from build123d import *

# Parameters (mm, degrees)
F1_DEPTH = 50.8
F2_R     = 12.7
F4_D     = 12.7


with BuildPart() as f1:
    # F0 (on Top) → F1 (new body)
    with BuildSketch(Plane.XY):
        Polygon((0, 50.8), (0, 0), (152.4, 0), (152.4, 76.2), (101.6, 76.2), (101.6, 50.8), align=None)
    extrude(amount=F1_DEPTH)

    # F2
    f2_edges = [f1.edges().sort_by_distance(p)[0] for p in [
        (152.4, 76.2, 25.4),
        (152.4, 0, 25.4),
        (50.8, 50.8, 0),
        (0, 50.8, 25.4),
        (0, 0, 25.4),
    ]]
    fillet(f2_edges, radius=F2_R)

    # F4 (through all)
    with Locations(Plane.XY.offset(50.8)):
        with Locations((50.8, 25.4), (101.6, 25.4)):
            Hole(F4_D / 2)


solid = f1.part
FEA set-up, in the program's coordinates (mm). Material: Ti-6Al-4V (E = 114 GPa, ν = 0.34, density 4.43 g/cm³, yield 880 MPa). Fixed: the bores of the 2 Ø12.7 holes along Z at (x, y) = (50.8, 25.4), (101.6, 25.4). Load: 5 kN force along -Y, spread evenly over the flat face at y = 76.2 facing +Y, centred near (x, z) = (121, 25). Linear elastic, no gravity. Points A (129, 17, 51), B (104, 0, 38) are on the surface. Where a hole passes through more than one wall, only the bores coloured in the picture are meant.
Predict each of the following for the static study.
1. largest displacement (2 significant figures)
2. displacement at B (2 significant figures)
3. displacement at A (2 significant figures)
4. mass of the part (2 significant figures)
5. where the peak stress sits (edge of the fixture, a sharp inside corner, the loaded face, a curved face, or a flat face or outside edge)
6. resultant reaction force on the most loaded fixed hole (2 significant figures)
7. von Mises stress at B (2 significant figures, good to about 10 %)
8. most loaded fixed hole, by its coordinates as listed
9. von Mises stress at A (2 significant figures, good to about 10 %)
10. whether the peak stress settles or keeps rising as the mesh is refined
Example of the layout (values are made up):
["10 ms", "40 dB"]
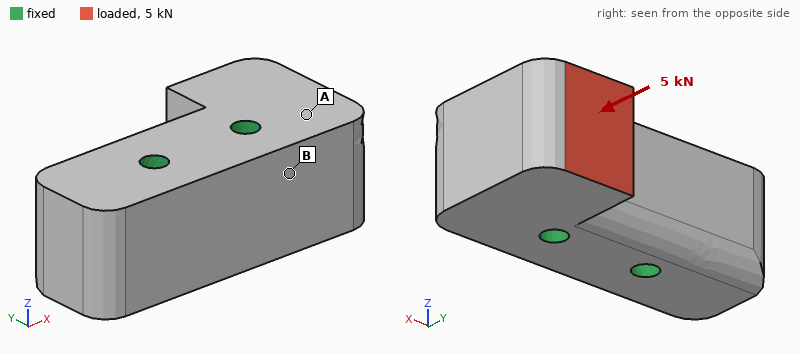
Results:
["4.2 µm", "0.85 µm", "1.8 µm", "1.9 kg", "edge of the fixture", "6.0 kN", "3.4 MPa", "(101.6, 25.4)", "1.5 MPa", "keeps rising"]
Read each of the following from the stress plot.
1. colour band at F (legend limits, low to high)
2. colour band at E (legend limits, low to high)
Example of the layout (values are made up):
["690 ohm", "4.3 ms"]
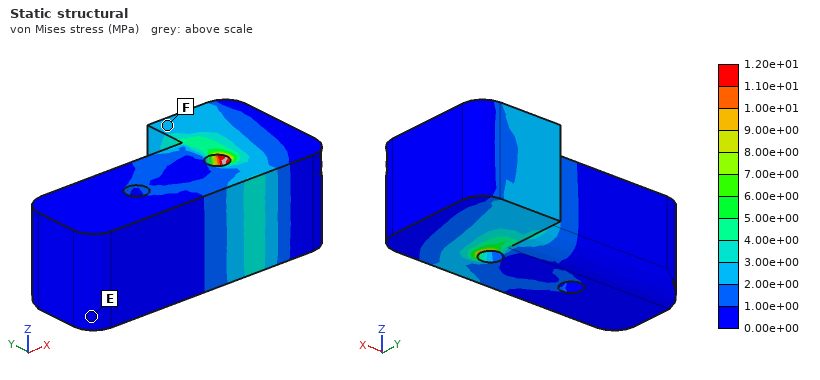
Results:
["2.00e+00 to 3.00e+00 MPa", "0.00e+00 to 1.00e+00 MPa"]
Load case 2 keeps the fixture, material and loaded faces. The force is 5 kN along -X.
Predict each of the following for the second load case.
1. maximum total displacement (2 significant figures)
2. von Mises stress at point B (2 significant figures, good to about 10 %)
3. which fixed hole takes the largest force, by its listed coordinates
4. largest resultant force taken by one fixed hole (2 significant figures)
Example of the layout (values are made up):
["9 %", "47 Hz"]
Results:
["12 µm", "7.2 MPa", "(101.6, 25.4)", "4.9 kN"]
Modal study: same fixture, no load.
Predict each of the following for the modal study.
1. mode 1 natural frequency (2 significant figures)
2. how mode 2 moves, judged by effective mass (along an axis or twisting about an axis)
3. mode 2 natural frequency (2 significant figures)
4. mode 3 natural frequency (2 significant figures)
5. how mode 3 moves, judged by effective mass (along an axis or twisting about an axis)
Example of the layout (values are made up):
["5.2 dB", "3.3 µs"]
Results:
["5700 Hz", "along Z", "7400 Hz", "8300 Hz", "along Y"]
